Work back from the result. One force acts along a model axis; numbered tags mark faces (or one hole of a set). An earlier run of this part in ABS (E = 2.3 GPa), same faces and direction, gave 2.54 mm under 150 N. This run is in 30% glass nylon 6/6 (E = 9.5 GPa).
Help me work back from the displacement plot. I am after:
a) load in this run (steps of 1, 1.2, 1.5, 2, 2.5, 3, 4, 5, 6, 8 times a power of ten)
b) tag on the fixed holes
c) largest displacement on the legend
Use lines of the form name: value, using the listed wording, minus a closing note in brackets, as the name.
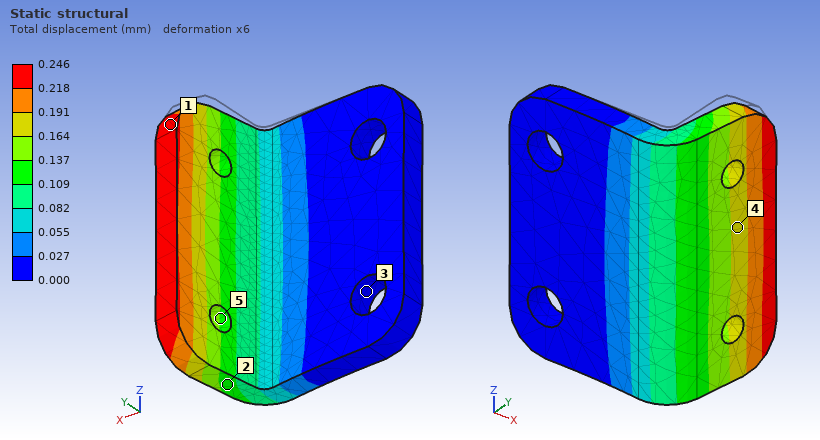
load in this run: 60 N
tag on the fixed holes: 3
largest displacement on the legend: 0.246 mm
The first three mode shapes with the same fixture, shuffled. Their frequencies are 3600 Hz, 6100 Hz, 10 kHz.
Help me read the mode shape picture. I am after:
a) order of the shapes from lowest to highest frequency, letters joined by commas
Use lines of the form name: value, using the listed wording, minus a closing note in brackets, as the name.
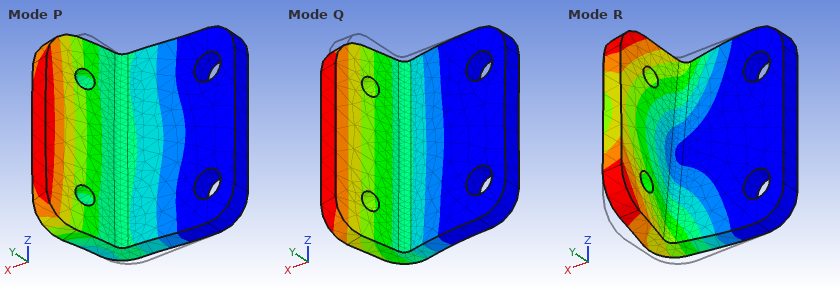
order of the shapes from lowest to highest frequency, letters joined by commas: Q, R, P
